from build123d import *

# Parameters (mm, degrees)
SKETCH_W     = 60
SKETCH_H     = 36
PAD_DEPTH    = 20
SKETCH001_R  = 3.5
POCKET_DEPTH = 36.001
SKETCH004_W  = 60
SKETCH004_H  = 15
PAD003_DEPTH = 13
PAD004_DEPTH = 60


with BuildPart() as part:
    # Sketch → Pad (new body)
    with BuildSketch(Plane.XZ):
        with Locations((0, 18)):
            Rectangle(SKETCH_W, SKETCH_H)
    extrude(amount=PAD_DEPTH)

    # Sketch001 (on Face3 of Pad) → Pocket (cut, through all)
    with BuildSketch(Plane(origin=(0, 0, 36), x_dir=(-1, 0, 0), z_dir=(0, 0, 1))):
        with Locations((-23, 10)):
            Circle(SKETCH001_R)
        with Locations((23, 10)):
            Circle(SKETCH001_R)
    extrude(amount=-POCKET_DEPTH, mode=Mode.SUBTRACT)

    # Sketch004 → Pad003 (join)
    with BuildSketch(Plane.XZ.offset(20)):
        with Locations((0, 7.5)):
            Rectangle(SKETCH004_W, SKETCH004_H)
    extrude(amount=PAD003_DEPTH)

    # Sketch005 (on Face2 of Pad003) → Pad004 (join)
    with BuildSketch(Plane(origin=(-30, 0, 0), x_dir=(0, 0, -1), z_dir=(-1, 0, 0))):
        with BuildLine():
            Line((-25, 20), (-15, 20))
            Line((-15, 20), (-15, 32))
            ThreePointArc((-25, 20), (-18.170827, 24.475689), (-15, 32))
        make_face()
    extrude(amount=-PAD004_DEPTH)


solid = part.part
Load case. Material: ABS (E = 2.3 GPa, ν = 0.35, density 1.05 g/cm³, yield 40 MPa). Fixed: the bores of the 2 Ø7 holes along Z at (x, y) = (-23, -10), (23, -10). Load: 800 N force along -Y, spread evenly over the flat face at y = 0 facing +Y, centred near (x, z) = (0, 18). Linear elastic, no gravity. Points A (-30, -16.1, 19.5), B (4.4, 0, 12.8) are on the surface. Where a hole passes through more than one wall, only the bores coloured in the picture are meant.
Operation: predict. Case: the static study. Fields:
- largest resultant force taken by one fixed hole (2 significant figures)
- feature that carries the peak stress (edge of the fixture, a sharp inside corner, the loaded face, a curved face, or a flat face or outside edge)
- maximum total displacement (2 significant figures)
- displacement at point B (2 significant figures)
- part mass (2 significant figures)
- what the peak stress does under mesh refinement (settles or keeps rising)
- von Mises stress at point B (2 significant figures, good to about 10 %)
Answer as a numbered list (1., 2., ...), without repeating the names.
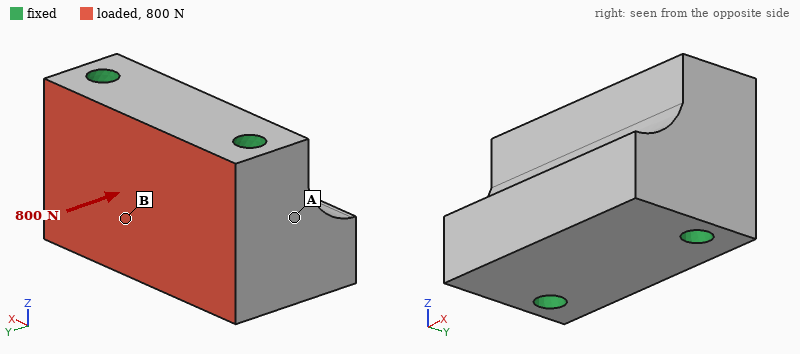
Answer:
1. 400 N
2. edge of the fixture
3. 11 µm
4. 7.3 µm
5. 57 g
6. keeps rising
7. 0.49 MPa
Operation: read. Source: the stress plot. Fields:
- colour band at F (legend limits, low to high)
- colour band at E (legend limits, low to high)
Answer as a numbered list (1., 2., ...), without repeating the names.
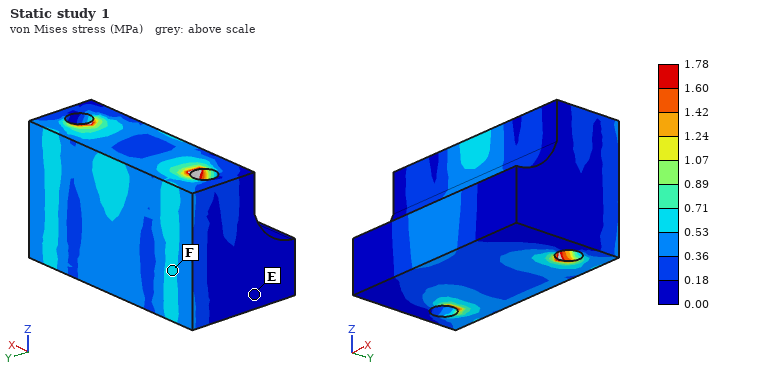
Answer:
1. 0.53 to 0.71 MPa
2. 0.00 to 0.18 MPa
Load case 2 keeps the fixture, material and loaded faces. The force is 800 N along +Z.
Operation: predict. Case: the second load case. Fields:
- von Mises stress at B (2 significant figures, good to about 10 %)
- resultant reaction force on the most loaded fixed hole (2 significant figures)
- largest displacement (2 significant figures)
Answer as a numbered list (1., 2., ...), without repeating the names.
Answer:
1. 0.76 MPa
2. 400 N
3. 20 µm
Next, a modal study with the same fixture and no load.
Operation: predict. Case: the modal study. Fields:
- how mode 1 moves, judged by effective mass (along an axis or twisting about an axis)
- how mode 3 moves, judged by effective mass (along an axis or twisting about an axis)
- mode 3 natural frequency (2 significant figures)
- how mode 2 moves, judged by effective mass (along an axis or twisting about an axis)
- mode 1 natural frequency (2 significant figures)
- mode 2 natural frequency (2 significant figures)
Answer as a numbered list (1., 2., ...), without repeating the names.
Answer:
1. along Z
2. along Z
3. 8900 Hz
4. along Y
5. 6600 Hz
6. 7500 Hz
